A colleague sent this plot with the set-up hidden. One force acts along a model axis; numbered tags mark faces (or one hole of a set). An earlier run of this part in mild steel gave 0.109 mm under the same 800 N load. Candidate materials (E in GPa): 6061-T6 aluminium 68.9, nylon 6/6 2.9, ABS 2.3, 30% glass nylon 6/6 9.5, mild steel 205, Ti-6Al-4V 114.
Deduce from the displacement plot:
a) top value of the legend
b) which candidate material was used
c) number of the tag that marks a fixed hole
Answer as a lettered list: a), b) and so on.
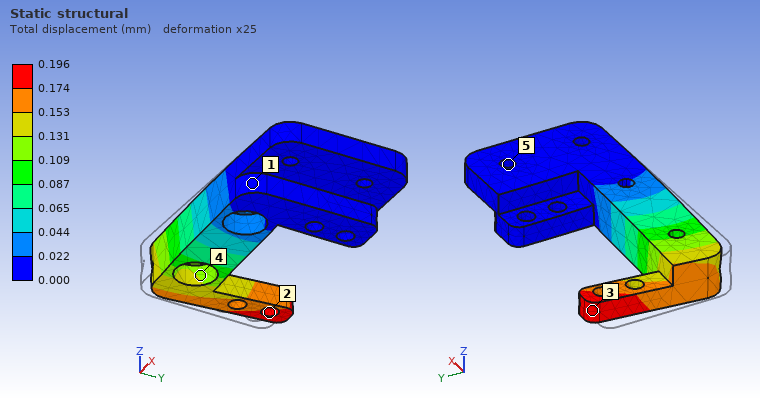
a) 0.196 mm
b) Ti-6Al-4V
c) 5
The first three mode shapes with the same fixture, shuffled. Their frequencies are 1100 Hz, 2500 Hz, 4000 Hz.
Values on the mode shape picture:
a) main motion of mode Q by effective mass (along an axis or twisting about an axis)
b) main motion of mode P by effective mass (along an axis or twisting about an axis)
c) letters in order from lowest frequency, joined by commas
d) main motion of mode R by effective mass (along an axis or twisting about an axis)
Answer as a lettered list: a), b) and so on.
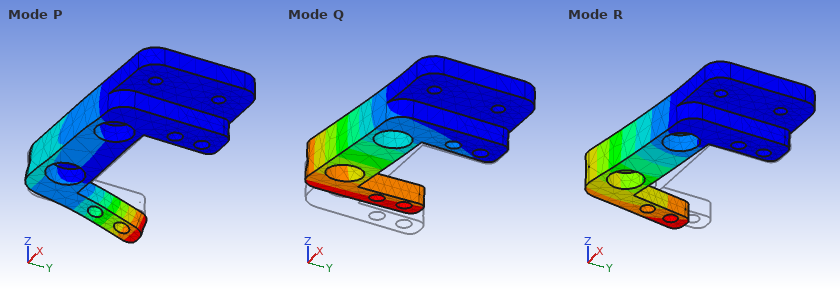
a) along Z
b) twisting about X
c) Q, R, P
d) along Y
